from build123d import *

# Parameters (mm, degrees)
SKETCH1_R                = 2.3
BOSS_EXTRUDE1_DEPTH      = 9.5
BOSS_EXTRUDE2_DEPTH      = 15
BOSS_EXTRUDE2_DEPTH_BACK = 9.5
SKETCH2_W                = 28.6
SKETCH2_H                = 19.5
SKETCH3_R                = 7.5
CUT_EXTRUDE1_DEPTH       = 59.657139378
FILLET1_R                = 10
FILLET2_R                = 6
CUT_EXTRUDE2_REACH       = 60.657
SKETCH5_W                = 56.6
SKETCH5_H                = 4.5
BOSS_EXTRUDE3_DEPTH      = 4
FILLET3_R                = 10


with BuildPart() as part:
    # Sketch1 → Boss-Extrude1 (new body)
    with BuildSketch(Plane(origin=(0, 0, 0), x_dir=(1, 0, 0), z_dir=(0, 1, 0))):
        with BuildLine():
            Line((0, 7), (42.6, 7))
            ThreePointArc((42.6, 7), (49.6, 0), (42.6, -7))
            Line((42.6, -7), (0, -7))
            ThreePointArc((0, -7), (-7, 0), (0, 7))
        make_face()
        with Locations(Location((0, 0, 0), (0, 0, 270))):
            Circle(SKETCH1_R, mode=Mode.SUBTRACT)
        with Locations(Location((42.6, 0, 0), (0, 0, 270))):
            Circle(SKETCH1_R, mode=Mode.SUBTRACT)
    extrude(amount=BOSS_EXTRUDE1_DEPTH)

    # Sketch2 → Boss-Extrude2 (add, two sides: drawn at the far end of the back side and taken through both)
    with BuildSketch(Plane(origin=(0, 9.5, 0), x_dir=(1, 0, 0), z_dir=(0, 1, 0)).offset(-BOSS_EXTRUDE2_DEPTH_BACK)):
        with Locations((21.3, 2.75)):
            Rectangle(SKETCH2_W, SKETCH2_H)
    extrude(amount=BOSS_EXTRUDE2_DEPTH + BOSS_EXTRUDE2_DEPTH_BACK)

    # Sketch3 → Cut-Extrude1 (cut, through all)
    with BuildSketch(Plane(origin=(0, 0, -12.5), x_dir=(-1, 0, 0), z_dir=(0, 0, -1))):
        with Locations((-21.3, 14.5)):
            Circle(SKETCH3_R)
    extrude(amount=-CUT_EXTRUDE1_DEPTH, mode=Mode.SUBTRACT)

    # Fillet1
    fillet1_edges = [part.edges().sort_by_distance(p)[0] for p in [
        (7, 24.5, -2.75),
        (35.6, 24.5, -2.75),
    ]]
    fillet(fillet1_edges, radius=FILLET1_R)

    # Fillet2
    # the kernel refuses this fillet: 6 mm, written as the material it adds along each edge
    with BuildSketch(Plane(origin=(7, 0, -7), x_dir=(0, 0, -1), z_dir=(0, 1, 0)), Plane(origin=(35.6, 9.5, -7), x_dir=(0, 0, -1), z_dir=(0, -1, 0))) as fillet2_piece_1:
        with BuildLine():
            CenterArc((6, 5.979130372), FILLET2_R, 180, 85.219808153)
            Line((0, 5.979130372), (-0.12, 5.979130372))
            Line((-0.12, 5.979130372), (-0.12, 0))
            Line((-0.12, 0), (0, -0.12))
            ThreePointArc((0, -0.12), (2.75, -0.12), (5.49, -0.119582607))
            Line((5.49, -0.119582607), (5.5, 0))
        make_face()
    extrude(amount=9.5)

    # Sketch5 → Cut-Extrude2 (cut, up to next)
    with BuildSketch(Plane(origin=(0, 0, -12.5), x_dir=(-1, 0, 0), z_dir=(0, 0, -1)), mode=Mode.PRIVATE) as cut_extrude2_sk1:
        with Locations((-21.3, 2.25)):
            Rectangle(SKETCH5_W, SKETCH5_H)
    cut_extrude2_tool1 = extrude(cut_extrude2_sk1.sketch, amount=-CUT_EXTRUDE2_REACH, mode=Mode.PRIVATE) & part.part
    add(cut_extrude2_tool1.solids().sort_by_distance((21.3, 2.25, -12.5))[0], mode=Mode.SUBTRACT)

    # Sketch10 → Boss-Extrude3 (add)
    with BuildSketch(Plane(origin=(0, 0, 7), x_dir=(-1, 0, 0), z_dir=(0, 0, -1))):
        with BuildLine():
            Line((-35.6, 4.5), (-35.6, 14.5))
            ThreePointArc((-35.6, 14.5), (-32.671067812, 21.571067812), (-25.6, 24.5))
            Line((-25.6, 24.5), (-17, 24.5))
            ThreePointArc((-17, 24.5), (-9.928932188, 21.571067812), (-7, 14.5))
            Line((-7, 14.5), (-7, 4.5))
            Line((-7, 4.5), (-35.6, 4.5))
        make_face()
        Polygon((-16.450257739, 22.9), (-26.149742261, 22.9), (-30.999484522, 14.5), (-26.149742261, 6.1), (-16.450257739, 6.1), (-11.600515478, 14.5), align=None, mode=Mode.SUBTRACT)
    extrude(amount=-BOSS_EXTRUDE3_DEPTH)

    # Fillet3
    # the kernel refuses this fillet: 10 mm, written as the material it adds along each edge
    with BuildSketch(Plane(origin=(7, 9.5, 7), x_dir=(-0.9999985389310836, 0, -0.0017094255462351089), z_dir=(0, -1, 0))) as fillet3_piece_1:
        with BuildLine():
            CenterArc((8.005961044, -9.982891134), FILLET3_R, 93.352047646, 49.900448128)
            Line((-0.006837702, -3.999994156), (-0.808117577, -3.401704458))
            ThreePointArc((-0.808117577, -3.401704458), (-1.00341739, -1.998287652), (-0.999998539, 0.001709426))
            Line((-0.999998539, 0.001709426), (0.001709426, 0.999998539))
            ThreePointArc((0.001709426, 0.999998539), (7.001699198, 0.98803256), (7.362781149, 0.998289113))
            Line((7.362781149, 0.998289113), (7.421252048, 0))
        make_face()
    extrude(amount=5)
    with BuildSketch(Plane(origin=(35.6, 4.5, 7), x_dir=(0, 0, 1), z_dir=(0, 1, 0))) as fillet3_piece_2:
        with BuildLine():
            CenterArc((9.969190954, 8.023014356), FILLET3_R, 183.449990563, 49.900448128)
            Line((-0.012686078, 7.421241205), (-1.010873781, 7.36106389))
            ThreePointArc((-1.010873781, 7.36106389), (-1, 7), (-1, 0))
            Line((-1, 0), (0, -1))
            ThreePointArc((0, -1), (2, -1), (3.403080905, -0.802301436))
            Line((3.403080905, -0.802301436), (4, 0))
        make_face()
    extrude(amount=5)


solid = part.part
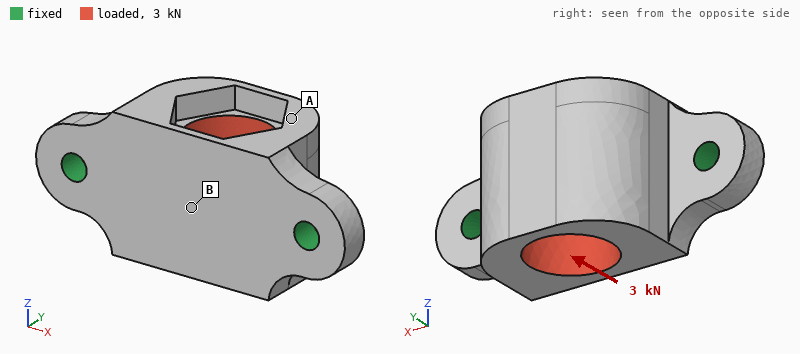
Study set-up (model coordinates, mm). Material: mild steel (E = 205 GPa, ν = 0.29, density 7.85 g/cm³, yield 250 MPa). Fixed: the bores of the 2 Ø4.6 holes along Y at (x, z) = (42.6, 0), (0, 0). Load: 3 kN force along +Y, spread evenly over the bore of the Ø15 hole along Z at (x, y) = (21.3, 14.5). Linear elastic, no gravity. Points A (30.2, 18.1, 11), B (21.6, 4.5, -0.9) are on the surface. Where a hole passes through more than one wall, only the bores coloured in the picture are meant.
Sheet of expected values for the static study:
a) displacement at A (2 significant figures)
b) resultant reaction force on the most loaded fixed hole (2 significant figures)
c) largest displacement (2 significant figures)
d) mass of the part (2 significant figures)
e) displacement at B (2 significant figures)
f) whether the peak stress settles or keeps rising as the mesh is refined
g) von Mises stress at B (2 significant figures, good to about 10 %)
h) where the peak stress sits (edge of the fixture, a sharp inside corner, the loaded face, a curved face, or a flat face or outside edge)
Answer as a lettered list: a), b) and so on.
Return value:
a) 6.4 µm
b) 1.5 kN
c) 17 µm
d) 77 g
e) 9.0 µm
f) keeps rising
g) 35 MPa
h) edge of the fixture
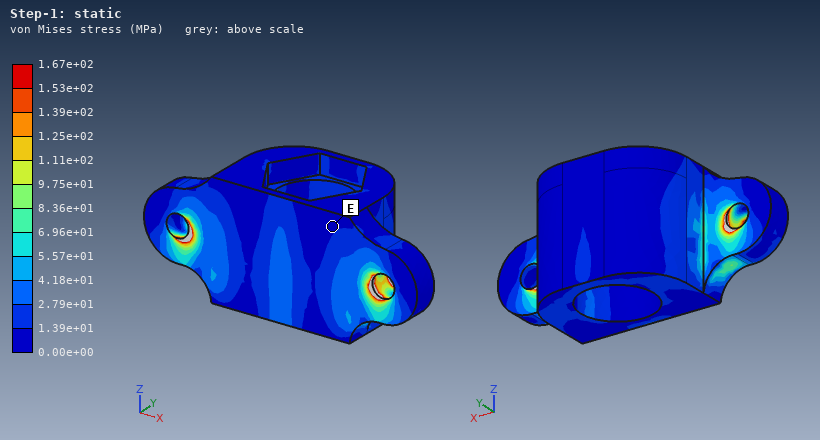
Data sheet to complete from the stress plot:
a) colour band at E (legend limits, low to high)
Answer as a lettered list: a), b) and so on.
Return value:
a) 0.00e+00 to 1.39e+01 MPa
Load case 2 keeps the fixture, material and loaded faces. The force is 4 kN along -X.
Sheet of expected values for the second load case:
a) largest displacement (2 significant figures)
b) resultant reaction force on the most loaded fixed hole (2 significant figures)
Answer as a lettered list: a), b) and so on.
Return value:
a) 8.3 µm
b) 2.2 kN
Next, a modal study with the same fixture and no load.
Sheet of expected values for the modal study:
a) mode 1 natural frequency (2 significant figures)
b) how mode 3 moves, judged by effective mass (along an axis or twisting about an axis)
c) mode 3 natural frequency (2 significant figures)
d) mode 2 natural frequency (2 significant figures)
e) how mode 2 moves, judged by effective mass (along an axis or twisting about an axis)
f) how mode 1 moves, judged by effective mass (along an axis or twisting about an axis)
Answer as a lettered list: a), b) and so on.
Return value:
a) 6500 Hz
b) along X
c) 17 kHz
d) 14 kHz
e) along Y
f) along Z
